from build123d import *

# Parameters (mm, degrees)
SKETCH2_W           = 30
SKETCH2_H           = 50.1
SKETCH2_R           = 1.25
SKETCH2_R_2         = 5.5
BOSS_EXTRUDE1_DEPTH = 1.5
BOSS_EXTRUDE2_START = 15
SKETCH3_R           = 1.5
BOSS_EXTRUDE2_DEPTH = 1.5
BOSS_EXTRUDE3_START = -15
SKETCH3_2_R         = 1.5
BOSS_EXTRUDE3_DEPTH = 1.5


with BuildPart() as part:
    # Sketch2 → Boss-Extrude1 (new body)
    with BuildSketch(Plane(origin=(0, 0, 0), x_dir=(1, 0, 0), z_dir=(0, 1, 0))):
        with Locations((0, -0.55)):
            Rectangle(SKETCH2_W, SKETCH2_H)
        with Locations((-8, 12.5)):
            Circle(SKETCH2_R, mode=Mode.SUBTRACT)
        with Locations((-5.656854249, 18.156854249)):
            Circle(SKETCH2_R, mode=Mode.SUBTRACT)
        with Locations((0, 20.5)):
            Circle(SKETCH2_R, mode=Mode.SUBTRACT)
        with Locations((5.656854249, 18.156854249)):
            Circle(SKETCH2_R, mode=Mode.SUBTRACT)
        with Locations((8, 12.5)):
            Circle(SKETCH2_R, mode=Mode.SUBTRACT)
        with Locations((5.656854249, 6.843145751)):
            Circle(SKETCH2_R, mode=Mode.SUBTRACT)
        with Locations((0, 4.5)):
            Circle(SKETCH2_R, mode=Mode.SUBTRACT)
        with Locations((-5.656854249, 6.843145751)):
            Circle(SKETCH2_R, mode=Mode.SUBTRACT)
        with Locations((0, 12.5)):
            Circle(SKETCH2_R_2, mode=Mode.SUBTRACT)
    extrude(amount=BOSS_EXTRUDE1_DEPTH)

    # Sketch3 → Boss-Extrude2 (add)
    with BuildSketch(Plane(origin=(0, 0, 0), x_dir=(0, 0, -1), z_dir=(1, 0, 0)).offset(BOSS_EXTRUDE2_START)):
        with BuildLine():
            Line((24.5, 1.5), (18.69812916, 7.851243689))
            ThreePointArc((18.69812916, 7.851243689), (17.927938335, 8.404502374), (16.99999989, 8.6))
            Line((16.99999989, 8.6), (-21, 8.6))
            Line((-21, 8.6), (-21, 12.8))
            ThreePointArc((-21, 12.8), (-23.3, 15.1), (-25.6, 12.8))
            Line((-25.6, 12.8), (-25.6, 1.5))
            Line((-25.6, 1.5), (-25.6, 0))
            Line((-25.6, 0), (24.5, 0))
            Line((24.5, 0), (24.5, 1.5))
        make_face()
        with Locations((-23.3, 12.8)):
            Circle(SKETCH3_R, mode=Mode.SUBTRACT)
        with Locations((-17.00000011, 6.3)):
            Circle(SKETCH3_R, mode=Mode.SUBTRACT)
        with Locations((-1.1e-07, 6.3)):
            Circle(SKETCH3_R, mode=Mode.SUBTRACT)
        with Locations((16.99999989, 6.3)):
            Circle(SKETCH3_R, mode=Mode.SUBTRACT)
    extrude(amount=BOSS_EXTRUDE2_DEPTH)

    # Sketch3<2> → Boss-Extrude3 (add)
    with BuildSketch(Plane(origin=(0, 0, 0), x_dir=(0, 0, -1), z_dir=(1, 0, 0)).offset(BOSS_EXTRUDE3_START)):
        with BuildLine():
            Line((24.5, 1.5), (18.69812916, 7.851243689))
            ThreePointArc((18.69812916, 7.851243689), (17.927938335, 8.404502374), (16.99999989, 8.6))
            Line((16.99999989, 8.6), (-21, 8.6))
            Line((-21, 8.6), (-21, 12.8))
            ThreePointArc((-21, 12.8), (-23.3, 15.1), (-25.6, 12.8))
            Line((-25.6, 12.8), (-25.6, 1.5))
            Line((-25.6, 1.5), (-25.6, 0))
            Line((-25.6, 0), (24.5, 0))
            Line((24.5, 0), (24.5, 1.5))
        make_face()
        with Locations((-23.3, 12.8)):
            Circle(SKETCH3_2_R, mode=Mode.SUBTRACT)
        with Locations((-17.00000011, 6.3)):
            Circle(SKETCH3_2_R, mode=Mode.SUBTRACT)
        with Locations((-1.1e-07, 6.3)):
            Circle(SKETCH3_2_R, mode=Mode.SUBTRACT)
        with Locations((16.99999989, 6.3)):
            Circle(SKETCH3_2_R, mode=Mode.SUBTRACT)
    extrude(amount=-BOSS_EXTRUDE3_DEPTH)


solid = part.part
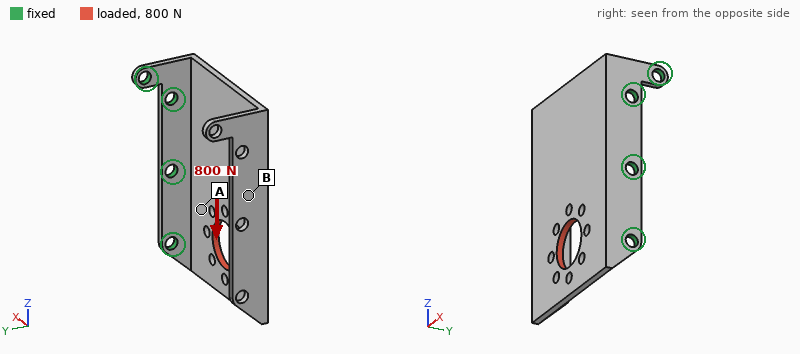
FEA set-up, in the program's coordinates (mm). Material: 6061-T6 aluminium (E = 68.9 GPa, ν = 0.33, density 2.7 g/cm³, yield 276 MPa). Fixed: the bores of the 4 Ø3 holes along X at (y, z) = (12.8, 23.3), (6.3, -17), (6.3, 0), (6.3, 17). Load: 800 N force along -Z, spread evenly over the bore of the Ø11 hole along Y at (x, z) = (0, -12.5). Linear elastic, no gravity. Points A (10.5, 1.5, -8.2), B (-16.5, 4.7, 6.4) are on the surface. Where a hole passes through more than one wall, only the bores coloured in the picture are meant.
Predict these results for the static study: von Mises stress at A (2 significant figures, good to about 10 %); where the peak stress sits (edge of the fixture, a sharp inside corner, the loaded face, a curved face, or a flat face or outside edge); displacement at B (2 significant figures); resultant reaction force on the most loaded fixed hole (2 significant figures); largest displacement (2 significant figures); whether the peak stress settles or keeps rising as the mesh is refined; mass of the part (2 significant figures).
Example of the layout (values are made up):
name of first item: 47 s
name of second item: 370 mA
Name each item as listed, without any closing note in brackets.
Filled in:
von Mises stress at A: 69 MPa
where the peak stress sits: edge of the fixture
displacement at B: 0.15 mm
resultant reaction force on the most loaded fixed hole: 440 N
largest displacement: 0.29 mm
whether the peak stress settles or keeps rising as the mesh is refined: keeps rising
mass of the part: 8.8 g
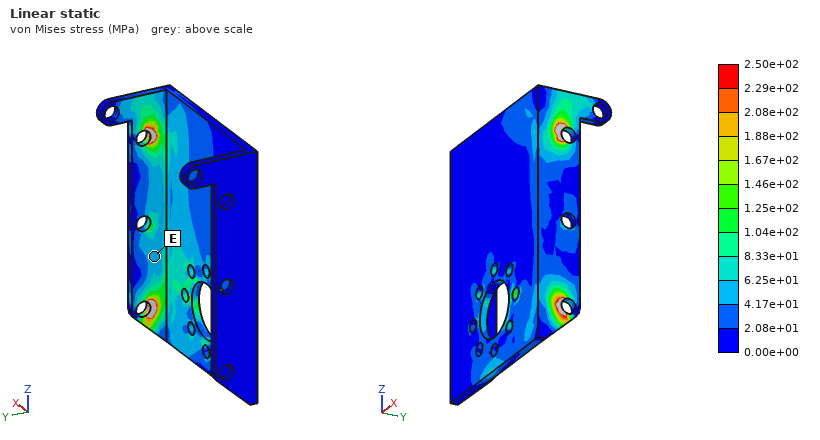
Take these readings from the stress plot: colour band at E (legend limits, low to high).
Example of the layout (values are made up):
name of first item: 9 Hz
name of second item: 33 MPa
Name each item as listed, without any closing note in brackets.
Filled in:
colour band at E: 4.17e+01 to 6.25e+01 MPa
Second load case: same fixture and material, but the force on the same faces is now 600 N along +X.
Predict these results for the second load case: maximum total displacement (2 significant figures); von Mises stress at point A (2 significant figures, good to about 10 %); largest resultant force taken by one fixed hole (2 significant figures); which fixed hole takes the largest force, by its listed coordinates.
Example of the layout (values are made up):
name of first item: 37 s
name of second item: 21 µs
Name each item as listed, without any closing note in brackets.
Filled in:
maximum total displacement: 0.43 mm
von Mises stress at point A: 29 MPa
largest resultant force taken by one fixed hole: 410 N
which fixed hole takes the largest force, by its listed coordinates: (6.3, -17)
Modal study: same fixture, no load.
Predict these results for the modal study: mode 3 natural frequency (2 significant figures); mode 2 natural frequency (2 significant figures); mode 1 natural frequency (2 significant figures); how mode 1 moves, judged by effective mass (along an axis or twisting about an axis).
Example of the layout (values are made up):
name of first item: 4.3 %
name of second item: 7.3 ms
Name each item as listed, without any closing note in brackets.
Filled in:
mode 3 natural frequency: 4100 Hz
mode 2 natural frequency: 1500 Hz
mode 1 natural frequency: 700 Hz
how mode 1 moves, judged by effective mass: along Y
